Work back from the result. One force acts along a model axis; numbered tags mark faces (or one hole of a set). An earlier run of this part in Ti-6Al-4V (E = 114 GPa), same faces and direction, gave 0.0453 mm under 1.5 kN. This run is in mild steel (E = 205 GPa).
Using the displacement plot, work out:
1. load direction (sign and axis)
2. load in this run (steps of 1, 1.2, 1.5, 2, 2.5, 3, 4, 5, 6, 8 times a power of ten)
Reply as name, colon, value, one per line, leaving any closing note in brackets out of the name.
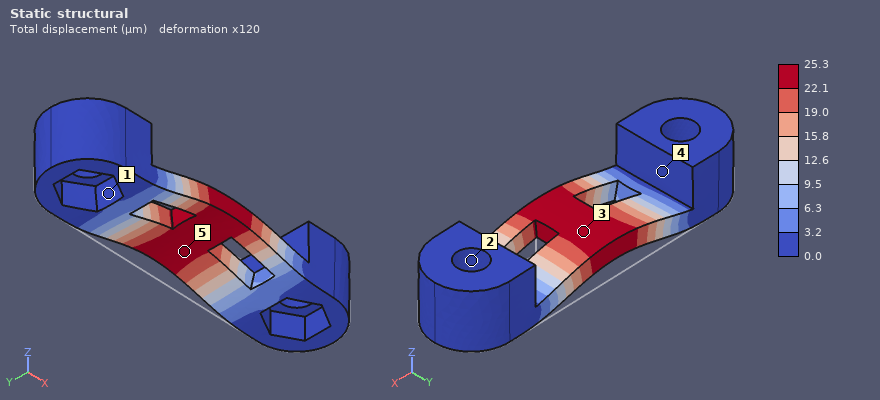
load direction: +Z
load in this run: 1.5 kN
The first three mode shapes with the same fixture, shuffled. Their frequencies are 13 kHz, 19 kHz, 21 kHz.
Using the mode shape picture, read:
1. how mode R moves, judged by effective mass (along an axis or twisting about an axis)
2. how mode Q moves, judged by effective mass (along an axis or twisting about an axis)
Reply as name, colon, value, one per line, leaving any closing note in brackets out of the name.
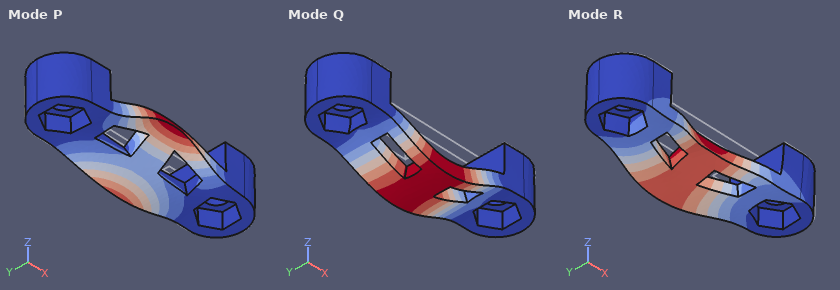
how mode R moves, judged by effective mass: along Y
how mode Q moves, judged by effective mass: along Z
